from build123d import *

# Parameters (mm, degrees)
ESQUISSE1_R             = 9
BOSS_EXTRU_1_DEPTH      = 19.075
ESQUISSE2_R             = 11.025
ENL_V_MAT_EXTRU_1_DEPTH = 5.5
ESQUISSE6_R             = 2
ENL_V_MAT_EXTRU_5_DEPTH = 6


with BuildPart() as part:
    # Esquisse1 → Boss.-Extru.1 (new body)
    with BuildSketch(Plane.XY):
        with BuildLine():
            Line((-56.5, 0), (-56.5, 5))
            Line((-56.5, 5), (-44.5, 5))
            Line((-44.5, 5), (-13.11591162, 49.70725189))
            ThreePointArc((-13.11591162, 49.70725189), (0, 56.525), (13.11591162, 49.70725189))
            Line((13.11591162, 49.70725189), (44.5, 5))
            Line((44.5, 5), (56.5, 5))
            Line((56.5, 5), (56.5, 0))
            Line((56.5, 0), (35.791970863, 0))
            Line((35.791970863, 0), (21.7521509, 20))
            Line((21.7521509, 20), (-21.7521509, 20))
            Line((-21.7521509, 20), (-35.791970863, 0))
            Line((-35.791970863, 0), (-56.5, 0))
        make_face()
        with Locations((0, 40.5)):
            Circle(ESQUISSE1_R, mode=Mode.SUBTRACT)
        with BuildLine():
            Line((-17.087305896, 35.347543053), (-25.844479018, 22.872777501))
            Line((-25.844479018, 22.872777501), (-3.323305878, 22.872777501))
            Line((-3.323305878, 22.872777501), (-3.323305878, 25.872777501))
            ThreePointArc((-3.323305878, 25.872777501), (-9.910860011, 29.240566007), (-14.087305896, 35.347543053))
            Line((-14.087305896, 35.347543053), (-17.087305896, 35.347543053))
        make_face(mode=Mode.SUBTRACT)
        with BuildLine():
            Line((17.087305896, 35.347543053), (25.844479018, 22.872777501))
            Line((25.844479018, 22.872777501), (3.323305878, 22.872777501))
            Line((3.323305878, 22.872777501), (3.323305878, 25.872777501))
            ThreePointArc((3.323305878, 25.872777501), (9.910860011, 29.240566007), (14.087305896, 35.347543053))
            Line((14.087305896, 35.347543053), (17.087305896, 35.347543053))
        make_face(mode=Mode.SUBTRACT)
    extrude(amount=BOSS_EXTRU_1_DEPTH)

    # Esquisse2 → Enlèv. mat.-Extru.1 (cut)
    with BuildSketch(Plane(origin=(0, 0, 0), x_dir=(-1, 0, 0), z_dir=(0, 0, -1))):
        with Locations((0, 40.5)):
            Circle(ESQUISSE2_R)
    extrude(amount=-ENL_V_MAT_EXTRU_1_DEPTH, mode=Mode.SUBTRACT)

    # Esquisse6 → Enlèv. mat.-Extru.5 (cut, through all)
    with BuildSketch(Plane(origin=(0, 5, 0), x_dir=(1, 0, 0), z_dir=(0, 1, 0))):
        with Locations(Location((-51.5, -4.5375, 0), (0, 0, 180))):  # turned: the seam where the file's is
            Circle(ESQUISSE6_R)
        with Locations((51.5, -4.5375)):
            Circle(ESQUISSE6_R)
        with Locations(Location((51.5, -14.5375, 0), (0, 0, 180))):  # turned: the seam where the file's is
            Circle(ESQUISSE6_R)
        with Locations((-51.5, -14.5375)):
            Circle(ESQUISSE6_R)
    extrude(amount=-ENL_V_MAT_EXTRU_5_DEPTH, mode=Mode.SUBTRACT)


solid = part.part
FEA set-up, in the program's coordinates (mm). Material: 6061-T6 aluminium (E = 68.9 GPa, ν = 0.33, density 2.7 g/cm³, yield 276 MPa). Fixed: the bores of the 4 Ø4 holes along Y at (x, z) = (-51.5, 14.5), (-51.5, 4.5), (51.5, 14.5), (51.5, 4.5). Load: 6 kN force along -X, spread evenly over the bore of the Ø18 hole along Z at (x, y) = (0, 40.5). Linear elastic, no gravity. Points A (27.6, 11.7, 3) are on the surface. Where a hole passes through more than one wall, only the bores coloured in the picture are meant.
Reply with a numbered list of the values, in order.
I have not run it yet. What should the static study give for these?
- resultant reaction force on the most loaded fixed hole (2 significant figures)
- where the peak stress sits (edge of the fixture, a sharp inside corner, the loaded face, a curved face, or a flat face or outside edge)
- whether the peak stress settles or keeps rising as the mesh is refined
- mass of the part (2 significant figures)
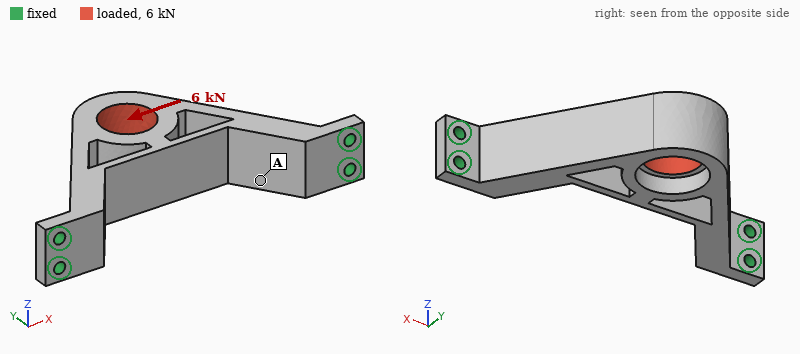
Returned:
1. 2.1 kN
2. edge of the fixture
3. keeps rising
4. 77 g
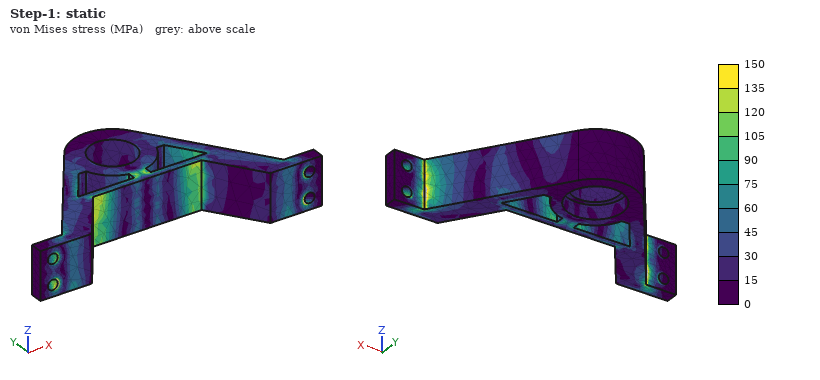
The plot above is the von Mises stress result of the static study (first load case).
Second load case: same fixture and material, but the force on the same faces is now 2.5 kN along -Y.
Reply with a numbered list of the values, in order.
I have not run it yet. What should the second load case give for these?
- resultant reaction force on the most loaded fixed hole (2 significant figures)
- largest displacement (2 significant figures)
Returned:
1. 1.1 kN
2. 76 µm
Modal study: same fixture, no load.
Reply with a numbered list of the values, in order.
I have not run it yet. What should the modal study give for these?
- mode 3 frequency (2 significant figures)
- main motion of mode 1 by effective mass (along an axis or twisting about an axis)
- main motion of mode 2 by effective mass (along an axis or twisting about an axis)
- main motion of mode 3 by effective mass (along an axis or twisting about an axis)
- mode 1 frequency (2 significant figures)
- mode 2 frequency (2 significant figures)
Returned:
1. 6500 Hz
2. along Z
3. along X
4. along Y
5. 1700 Hz
6. 4500 Hz
